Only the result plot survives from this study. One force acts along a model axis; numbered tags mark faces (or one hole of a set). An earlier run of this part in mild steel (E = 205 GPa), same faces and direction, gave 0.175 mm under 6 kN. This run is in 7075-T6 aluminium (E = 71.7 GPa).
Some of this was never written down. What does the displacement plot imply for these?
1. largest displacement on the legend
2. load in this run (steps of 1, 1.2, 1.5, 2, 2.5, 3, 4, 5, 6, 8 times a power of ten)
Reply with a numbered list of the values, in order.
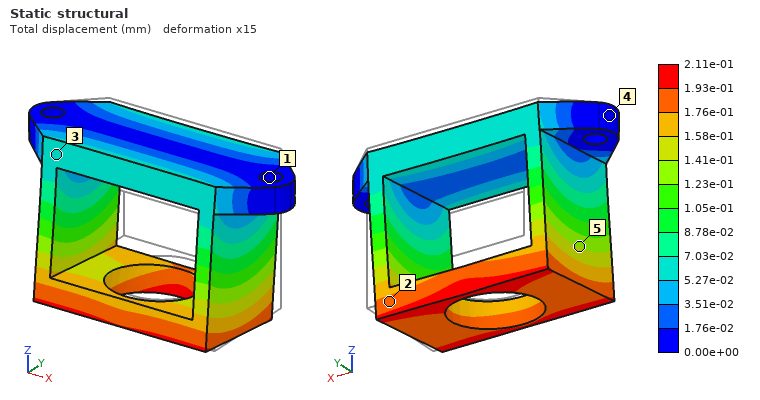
1. 2.11e-01 mm
2. 2.5 kN
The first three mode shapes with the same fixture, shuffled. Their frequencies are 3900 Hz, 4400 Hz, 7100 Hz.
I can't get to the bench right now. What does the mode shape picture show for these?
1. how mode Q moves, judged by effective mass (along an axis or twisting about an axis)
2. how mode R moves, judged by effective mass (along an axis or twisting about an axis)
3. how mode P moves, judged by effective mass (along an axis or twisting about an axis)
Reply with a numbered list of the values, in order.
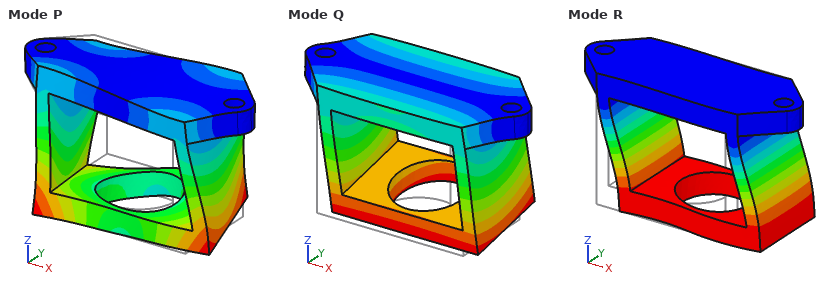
1. along Y
2. along X
3. twisting about Z
